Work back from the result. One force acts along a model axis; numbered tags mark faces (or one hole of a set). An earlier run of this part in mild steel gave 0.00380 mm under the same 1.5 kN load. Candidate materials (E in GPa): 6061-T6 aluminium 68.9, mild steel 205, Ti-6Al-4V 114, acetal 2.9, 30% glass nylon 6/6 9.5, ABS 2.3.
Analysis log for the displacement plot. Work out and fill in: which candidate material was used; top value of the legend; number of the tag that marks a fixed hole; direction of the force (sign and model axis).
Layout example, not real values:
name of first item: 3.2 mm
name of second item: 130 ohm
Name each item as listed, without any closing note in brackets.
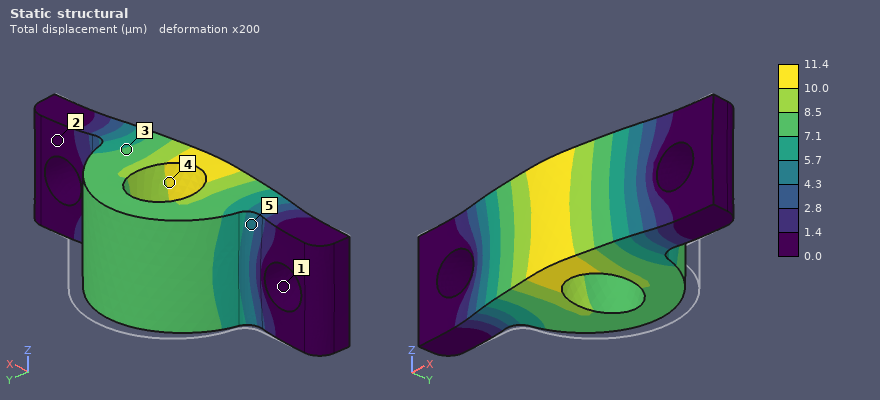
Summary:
which candidate material was used: 6061-T6 aluminium
top value of the legend: 11.4 µm
number of the tag that marks a fixed hole: 1
direction of the force: -Y
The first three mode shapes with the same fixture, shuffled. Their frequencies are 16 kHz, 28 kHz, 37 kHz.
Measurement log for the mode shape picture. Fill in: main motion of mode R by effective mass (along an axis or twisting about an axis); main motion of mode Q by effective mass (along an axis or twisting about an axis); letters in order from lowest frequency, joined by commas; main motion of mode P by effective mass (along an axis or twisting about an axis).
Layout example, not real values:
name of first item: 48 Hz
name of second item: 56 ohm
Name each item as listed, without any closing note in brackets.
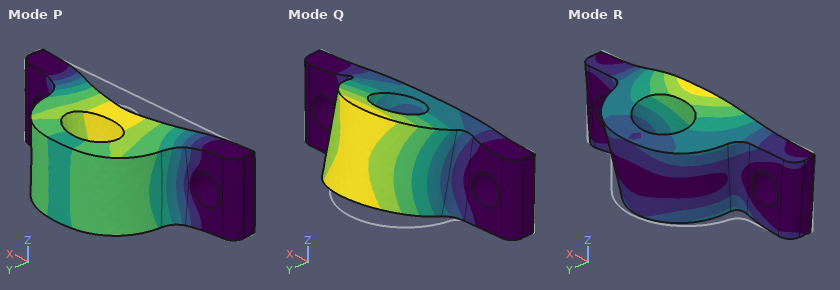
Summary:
main motion of mode R by effective mass: along Z
main motion of mode Q by effective mass: along Z
letters in order from lowest frequency, joined by commas: Q, P, R
main motion of mode P by effective mass: along Y
